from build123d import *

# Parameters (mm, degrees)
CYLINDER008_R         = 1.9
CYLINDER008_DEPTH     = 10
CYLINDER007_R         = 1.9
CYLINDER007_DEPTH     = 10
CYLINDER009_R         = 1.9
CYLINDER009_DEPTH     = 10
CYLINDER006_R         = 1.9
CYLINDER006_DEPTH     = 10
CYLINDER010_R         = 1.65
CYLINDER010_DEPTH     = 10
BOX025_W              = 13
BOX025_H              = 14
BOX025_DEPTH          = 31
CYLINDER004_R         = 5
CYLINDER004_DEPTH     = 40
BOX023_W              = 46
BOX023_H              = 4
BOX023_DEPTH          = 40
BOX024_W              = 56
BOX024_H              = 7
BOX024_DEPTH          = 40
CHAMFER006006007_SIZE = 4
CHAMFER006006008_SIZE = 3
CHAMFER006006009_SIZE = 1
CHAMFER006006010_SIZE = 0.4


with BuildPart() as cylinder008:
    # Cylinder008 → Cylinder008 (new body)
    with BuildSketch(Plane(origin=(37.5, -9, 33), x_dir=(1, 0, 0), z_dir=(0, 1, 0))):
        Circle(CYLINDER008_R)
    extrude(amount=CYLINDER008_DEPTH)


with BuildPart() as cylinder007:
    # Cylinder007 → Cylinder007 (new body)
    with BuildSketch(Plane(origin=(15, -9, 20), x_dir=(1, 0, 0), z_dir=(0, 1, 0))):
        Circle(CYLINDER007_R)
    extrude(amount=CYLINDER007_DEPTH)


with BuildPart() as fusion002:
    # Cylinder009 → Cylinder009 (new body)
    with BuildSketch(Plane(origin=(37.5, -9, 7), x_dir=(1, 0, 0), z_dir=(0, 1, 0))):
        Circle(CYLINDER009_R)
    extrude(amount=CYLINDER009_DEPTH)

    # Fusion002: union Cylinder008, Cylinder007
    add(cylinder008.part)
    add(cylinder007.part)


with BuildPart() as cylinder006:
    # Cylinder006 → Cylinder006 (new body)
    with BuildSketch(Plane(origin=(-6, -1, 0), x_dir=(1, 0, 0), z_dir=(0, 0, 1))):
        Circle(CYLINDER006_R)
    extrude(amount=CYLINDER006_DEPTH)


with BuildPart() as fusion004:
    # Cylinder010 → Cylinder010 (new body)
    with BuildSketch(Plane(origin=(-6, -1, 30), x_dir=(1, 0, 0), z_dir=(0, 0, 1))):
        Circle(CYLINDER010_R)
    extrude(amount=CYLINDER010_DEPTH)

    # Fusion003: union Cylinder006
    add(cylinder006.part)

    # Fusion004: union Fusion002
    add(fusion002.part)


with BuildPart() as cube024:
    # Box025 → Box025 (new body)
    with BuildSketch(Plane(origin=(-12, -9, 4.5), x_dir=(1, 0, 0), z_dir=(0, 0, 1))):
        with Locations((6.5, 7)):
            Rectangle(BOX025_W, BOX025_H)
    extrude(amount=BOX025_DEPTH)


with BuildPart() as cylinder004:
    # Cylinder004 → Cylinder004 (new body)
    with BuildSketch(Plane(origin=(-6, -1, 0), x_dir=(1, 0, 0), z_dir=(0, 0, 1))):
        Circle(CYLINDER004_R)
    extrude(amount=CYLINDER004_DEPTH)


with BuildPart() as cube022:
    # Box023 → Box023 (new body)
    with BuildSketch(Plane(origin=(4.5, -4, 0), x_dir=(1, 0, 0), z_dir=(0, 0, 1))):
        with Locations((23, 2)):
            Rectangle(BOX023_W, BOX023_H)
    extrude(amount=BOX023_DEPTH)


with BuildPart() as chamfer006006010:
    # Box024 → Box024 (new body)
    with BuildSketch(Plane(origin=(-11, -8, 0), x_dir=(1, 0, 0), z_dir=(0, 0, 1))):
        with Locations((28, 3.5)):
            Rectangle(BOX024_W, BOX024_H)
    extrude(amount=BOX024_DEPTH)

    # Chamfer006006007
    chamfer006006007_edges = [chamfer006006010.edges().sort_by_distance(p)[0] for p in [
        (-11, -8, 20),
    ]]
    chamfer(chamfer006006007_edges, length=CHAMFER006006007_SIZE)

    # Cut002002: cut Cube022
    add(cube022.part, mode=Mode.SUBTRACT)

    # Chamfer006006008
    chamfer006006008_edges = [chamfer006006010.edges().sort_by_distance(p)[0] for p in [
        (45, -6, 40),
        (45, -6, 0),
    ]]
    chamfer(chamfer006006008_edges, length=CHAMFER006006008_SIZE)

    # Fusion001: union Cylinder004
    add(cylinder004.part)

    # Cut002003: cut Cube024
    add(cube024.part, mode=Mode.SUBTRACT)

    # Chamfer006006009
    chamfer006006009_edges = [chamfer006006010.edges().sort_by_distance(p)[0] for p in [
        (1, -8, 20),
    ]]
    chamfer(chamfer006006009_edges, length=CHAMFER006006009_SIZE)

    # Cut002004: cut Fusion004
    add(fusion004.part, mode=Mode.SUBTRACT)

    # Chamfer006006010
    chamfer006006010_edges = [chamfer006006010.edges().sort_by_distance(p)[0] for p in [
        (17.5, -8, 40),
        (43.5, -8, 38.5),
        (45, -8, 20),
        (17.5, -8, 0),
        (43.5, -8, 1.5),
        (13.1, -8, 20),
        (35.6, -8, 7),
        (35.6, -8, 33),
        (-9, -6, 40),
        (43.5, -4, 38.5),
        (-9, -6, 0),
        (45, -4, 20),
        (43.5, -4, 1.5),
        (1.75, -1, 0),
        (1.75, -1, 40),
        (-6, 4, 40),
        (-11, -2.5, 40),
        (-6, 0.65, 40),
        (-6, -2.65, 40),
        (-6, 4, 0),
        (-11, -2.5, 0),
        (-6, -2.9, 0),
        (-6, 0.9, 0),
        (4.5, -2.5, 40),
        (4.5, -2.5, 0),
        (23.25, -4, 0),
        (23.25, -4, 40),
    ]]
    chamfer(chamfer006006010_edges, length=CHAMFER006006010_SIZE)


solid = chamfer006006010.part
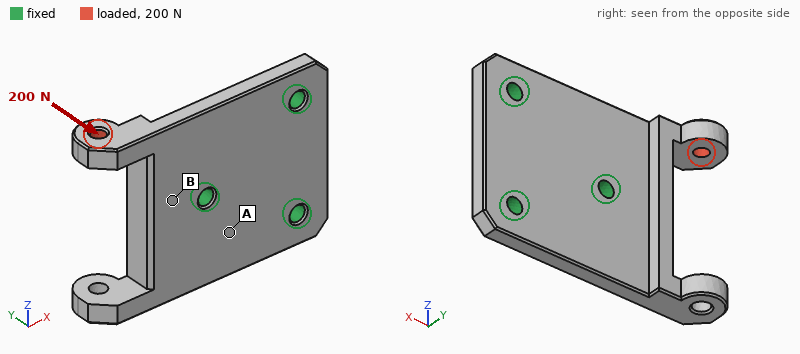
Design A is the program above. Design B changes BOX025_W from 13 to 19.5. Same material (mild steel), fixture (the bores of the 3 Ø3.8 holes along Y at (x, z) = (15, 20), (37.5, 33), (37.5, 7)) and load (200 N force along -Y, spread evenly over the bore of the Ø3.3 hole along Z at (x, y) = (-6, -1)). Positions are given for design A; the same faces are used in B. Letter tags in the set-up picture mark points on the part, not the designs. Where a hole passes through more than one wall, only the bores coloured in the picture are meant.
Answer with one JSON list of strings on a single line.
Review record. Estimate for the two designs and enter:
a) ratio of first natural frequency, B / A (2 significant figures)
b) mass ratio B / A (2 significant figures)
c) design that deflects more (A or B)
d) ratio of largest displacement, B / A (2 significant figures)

["0.85", "0.91", "B", "1.7"]
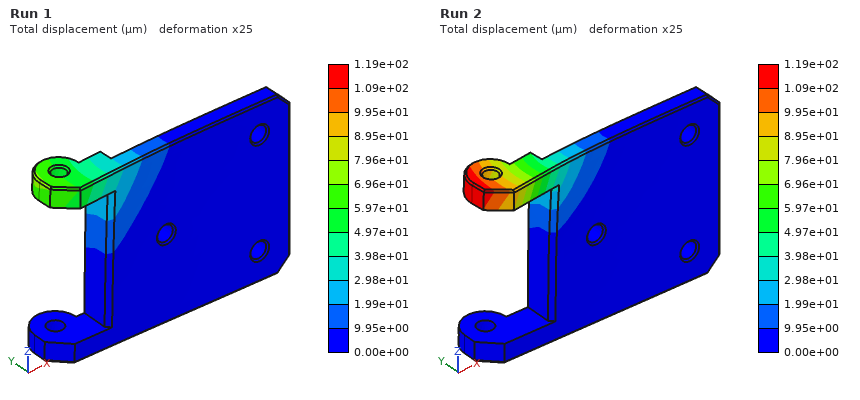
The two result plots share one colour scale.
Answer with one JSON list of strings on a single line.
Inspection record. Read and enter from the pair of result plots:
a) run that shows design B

["Run 2"]
